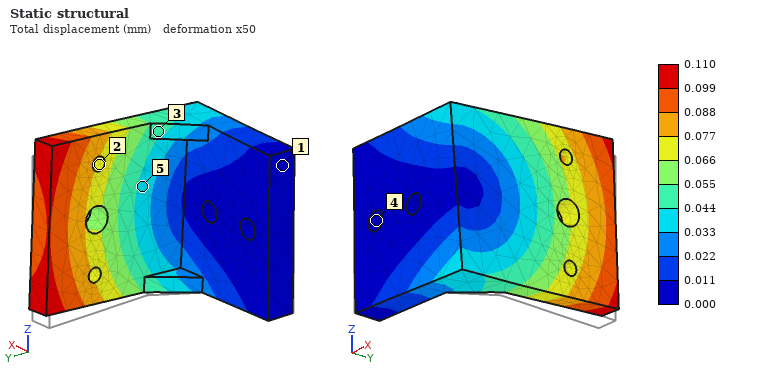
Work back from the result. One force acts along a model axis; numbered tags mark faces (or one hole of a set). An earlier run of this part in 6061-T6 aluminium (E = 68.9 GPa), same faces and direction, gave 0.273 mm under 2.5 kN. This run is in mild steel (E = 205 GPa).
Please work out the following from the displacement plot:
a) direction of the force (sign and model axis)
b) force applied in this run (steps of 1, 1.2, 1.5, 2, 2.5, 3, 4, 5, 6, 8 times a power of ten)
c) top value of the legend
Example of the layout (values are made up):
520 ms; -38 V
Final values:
+Z; 3 kN; 0.110 mm
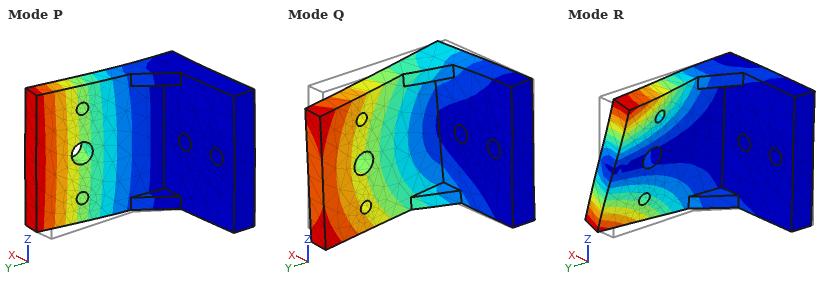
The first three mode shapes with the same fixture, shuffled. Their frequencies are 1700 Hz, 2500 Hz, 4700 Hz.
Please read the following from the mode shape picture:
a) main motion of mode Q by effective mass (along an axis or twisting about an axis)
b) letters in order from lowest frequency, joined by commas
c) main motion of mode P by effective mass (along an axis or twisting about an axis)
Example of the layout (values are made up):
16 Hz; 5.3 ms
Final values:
along Z; P, Q, R; along X
